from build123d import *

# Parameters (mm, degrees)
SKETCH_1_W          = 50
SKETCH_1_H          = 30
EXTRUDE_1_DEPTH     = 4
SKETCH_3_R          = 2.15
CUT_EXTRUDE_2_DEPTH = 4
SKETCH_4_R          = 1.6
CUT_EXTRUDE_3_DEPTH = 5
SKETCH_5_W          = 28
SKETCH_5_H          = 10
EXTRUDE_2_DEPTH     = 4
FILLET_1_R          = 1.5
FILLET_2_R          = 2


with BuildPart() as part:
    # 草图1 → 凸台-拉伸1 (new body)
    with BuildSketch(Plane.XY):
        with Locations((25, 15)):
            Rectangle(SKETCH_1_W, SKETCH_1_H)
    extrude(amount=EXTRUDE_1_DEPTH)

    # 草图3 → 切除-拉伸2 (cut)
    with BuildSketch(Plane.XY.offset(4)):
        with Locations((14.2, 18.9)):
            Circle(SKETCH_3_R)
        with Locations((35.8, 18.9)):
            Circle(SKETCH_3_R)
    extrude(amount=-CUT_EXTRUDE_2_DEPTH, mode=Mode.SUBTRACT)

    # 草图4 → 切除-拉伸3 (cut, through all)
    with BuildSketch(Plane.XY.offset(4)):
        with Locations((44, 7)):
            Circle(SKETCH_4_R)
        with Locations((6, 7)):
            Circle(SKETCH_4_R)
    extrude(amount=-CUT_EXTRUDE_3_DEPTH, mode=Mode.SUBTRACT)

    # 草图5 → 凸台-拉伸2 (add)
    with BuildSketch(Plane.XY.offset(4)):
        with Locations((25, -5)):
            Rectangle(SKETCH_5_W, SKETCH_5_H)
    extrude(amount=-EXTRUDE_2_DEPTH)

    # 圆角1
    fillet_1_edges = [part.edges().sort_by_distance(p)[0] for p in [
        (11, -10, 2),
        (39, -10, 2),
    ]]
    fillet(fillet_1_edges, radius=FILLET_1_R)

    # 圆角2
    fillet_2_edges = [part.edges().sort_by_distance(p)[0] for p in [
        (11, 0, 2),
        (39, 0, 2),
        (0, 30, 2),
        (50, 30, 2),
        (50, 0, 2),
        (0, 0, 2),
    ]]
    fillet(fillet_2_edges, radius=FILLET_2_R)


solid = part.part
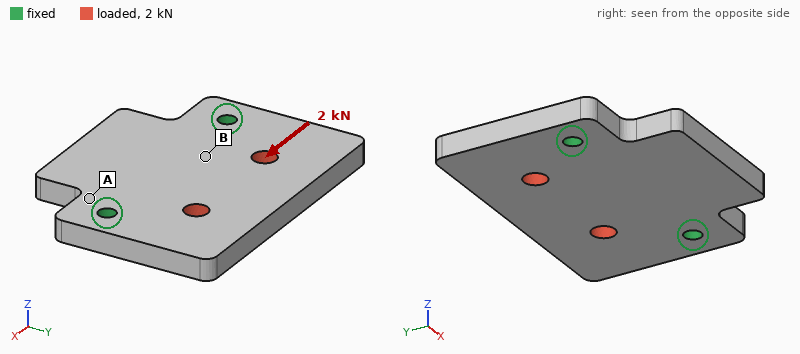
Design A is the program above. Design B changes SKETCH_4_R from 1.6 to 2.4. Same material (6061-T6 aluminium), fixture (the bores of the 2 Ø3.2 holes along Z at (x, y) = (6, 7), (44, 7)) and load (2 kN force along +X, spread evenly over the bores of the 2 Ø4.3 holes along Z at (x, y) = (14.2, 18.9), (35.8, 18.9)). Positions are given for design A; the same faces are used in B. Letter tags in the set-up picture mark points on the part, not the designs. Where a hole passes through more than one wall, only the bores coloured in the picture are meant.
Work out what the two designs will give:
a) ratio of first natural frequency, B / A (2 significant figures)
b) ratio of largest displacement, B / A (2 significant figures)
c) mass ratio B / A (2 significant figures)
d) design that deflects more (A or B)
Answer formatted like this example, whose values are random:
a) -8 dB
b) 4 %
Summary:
a) 1.1
b) 0.88
c) 0.99
d) A
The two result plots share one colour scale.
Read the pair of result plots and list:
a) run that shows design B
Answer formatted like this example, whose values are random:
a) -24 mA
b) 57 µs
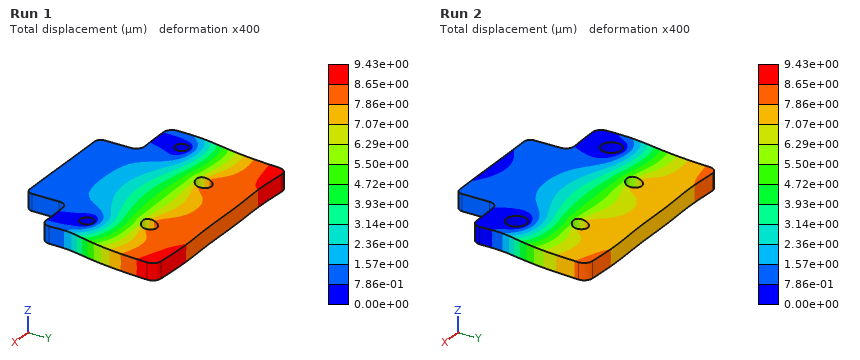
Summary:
a) Run 2
